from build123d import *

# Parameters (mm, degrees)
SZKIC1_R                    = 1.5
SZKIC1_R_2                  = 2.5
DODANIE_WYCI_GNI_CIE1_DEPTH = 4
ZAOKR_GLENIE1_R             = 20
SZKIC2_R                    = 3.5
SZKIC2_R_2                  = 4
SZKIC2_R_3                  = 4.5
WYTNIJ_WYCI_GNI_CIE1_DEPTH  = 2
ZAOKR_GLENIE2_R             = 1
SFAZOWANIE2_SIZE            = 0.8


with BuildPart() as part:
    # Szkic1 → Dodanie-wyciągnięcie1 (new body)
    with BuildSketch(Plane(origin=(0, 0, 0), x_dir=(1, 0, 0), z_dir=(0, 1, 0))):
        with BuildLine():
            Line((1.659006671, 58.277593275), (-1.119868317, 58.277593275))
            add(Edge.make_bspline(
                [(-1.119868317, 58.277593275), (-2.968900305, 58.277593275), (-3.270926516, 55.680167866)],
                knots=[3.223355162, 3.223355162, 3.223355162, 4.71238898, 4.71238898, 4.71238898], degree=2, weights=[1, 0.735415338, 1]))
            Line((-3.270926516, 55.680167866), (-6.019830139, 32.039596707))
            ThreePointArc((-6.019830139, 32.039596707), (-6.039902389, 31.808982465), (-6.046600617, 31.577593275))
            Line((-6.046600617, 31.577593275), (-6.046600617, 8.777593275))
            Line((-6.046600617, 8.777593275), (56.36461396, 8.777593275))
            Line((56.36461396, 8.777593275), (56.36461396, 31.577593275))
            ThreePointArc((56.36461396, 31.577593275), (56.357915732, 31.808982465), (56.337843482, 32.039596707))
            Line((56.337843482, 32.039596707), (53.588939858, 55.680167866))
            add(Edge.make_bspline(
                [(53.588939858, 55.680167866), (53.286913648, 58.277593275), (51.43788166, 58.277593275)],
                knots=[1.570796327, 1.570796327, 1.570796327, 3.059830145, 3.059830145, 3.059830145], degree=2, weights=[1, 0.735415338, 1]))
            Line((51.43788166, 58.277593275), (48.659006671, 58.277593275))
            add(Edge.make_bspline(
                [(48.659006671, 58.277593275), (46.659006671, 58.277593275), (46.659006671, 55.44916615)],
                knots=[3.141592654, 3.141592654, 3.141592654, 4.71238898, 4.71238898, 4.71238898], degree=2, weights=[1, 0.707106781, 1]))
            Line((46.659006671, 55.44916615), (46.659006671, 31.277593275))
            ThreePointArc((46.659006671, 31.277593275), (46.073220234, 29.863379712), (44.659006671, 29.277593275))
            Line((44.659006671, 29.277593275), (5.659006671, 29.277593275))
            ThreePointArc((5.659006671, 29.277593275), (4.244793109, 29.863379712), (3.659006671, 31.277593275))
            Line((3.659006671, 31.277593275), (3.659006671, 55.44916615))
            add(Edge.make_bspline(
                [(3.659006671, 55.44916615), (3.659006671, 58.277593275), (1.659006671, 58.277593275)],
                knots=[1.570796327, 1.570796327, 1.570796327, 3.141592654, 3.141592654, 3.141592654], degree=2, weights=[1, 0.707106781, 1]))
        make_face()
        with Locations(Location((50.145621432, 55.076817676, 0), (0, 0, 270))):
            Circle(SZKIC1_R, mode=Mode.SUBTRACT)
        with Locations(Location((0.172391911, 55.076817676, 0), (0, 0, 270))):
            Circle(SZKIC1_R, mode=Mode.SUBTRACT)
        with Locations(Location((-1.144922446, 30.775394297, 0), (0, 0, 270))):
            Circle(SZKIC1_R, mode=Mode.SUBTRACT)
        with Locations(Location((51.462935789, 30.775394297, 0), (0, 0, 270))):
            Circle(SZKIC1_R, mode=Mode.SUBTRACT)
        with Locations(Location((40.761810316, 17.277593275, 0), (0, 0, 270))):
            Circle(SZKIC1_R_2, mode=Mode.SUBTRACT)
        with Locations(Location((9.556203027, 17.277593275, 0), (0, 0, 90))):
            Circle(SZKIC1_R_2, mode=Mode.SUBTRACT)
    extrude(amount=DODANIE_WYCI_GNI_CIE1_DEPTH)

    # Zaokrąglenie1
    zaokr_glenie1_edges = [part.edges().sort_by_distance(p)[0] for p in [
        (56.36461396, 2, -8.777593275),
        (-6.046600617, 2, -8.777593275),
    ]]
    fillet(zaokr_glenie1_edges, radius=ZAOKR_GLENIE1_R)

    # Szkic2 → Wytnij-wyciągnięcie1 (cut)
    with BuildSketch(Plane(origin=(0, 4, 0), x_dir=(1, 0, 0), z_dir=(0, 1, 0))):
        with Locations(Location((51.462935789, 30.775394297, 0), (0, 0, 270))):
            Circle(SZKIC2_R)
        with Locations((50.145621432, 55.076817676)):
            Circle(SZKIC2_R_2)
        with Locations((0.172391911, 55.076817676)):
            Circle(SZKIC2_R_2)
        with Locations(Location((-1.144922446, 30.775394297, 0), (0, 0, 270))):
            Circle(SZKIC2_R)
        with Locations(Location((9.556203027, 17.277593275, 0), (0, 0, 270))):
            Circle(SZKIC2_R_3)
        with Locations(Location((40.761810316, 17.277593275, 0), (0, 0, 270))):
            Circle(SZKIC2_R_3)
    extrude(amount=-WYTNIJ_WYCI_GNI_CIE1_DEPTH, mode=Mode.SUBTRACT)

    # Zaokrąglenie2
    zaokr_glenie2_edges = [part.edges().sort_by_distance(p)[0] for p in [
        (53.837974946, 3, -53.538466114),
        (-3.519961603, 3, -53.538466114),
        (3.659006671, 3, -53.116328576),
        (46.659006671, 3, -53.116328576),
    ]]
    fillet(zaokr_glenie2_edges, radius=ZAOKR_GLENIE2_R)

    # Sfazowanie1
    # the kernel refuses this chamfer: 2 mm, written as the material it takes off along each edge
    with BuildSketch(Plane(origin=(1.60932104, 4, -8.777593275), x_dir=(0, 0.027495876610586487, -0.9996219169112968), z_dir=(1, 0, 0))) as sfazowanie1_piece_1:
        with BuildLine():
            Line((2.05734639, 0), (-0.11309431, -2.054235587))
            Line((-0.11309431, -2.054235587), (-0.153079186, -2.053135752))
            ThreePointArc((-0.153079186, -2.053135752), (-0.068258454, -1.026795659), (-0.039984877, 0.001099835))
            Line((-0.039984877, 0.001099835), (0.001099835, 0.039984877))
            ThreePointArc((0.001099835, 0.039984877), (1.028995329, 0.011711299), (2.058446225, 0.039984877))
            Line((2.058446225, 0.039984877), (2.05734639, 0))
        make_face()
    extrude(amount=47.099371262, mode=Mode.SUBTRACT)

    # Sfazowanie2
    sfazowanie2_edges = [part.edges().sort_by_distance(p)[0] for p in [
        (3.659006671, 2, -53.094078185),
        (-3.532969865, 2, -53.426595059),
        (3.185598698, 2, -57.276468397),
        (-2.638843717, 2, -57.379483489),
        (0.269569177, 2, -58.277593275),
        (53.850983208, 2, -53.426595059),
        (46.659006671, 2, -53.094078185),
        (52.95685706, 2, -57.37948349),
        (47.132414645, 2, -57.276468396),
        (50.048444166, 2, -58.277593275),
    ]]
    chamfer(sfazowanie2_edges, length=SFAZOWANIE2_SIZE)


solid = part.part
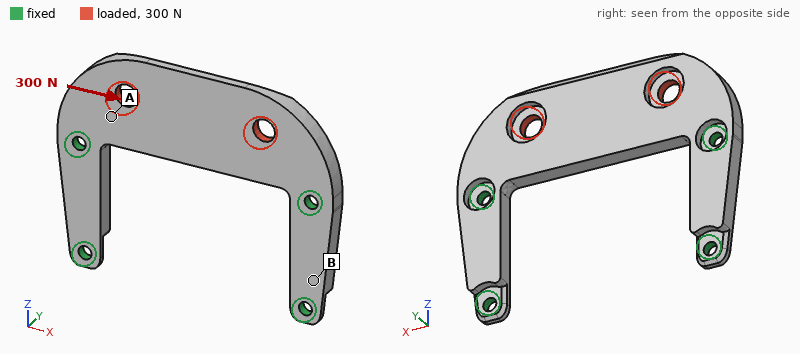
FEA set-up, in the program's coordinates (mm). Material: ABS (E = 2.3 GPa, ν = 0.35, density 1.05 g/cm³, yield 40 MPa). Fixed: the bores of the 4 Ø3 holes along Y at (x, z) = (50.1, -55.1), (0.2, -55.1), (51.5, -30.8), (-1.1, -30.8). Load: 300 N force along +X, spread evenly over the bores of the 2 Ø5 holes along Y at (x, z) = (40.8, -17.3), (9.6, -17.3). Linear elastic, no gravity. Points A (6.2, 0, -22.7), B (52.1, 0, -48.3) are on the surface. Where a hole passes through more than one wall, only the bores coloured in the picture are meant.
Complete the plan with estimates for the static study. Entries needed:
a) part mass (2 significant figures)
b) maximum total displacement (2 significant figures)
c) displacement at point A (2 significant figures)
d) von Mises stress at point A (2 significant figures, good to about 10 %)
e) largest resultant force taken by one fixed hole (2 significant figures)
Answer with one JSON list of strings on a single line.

["5.8 g", "0.11 mm", "0.068 mm", "4.9 MPa", "170 N"]
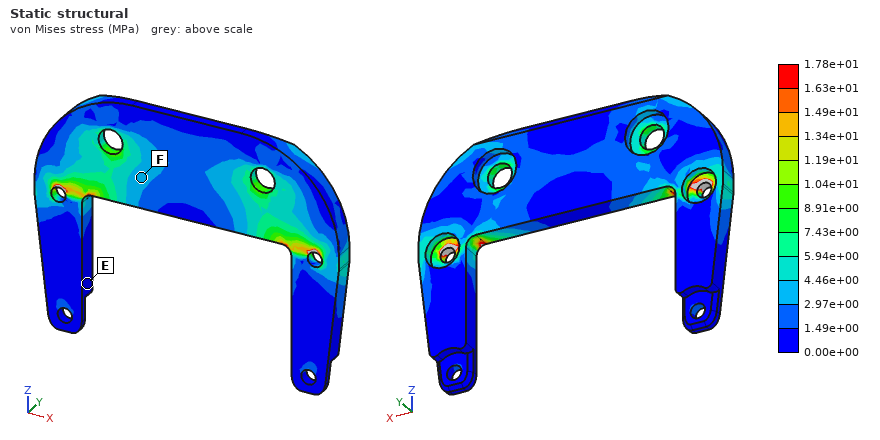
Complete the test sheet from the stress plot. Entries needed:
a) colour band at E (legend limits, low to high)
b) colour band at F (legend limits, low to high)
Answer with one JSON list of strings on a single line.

["0.00e+00 to 1.49e+00 MPa", "2.97e+00 to 4.46e+00 MPa"]
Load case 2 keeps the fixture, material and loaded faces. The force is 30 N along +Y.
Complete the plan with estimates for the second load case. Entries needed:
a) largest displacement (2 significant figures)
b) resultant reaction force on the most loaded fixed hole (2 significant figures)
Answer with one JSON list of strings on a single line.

["0.48 mm", "23 N"]
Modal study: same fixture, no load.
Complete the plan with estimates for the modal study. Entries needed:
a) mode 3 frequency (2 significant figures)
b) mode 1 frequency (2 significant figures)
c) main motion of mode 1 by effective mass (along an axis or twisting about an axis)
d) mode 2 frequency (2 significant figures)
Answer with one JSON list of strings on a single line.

["2400 Hz", "870 Hz", "along Y", "2400 Hz"]
